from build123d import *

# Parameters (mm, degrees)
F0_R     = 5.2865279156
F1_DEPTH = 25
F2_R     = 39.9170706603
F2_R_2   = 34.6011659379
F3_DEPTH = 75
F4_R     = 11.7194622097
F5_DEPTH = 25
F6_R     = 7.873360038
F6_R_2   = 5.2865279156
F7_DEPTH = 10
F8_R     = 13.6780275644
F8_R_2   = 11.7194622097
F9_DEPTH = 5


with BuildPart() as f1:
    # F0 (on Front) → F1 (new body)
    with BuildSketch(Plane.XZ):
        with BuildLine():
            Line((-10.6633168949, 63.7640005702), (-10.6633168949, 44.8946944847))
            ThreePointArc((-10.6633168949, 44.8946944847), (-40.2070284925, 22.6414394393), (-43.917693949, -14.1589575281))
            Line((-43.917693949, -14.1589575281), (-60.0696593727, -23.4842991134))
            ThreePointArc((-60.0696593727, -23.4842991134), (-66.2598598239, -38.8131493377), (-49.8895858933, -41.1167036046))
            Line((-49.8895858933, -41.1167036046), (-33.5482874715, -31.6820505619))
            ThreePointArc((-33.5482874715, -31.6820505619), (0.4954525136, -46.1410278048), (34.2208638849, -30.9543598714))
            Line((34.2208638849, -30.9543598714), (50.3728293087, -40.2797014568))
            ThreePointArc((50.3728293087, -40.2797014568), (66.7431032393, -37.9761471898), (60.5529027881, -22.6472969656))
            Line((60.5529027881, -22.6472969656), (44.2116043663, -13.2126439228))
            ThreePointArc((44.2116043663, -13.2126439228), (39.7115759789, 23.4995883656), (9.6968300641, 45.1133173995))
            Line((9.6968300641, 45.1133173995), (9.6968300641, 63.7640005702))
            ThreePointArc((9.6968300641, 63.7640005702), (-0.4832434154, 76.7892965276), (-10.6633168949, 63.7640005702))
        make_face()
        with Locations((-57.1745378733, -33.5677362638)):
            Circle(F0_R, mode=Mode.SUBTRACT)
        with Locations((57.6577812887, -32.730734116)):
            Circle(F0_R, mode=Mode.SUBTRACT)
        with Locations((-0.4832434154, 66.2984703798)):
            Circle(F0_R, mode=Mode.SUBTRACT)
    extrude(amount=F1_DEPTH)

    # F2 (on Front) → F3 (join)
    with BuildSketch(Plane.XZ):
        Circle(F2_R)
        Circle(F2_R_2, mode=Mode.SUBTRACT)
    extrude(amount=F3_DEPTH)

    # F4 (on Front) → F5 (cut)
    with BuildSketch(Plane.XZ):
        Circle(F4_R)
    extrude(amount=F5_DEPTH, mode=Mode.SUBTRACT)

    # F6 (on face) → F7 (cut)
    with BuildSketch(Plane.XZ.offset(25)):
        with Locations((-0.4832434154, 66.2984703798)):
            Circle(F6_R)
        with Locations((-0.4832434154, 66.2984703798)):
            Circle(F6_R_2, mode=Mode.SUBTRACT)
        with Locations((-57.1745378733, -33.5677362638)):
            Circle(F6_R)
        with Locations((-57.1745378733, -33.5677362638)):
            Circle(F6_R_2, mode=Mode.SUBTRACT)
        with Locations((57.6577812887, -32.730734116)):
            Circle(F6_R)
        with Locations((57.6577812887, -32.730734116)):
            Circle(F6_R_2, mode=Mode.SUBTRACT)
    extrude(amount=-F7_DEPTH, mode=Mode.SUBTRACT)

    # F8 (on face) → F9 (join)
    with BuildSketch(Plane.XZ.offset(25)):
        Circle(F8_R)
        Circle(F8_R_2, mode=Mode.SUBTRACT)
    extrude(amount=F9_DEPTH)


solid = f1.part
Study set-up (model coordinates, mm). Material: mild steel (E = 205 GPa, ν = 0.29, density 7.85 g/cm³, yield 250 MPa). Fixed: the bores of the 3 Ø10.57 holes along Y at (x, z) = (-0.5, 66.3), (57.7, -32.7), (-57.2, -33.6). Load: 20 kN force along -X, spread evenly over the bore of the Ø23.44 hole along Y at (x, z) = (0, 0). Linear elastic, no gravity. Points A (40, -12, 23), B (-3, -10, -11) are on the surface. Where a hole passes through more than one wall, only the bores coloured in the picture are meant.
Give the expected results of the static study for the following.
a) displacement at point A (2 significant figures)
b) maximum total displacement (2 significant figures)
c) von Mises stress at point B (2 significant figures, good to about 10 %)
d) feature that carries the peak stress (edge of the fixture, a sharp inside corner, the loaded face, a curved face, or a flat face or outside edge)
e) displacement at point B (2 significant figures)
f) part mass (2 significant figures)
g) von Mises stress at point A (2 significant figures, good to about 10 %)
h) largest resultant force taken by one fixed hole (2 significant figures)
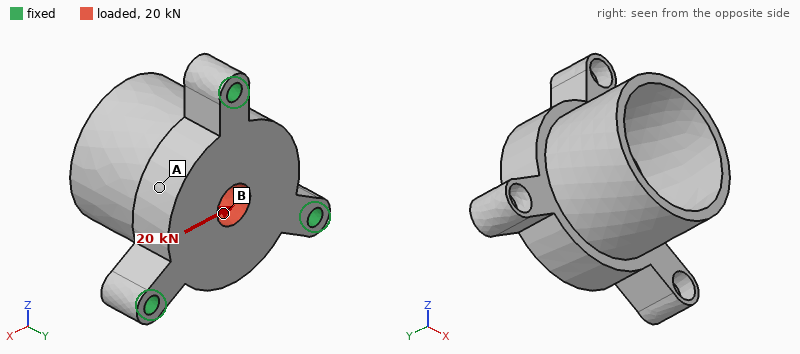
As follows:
5.9 µm
11 µm
20 MPa
edge of the fixture
4.8 µm
2.0 kg
6.7 MPa
9.2 kN
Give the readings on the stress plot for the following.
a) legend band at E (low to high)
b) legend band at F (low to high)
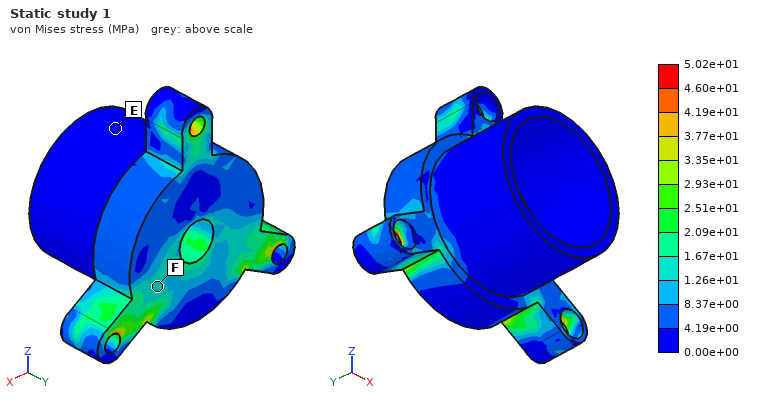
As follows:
0.00e+00 to 4.19e+00 MPa
1.26e+01 to 1.67e+01 MPa
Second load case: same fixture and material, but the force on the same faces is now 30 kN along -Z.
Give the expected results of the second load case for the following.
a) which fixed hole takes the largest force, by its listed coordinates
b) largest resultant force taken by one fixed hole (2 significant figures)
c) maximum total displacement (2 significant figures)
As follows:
(-0.5, 66.3)
16 kN
18 µm
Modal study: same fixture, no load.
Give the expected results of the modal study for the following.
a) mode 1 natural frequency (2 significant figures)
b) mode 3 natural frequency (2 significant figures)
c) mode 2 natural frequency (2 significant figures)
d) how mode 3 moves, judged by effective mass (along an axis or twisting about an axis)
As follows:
4100 Hz
4700 Hz
4100 Hz
along Y
